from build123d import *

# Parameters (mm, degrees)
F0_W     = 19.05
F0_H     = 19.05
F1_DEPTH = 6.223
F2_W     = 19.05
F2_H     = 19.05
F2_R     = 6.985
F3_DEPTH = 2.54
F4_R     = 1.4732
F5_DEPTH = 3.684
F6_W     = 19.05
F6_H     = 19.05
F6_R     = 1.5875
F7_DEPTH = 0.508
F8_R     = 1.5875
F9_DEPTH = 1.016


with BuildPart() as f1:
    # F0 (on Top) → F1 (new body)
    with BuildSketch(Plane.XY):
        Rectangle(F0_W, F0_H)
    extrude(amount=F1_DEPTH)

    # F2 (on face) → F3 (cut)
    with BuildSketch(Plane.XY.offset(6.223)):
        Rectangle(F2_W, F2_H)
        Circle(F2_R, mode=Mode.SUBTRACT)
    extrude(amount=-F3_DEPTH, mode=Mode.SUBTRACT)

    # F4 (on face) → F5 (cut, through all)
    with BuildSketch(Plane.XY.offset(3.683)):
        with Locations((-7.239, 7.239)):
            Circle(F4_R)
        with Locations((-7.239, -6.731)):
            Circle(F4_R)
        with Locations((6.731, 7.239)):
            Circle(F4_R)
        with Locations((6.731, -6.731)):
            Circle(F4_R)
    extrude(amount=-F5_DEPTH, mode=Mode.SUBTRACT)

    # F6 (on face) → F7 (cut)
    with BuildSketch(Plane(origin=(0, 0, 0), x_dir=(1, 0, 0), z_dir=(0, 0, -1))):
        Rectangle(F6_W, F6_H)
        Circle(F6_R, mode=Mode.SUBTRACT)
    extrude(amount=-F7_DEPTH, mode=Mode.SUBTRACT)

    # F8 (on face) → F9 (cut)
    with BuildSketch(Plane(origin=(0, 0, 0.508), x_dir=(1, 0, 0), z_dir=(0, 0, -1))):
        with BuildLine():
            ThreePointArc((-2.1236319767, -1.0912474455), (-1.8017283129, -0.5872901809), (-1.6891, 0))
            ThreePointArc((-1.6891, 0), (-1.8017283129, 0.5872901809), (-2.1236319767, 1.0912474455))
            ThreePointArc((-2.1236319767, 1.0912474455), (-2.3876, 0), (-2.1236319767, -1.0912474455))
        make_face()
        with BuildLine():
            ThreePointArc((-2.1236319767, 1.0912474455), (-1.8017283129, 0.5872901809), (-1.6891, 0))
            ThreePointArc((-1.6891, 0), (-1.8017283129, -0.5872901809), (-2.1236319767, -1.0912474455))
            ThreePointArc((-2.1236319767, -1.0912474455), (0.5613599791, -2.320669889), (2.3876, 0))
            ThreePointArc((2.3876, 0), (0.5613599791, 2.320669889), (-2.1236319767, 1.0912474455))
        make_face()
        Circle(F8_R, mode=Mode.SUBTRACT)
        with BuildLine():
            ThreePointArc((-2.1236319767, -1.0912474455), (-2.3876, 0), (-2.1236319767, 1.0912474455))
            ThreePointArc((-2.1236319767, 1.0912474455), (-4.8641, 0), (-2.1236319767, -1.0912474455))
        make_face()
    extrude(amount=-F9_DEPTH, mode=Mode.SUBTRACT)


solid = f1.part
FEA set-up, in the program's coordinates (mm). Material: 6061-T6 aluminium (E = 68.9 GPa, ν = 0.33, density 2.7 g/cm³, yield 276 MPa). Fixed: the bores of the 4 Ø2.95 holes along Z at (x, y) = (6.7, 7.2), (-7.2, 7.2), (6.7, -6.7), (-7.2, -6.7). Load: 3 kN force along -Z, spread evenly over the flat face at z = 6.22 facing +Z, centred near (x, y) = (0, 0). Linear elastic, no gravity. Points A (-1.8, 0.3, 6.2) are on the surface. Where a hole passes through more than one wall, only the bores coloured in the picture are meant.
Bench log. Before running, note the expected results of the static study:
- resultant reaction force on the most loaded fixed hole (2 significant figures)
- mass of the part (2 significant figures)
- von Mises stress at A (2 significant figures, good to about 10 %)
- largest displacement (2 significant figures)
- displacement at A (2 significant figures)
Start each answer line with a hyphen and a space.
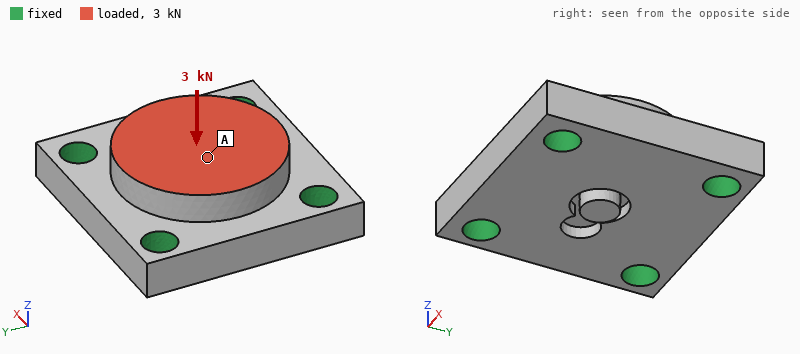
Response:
- 870 N
- 3.9 g
- 26 MPa
- 10 µm
- 10 µm
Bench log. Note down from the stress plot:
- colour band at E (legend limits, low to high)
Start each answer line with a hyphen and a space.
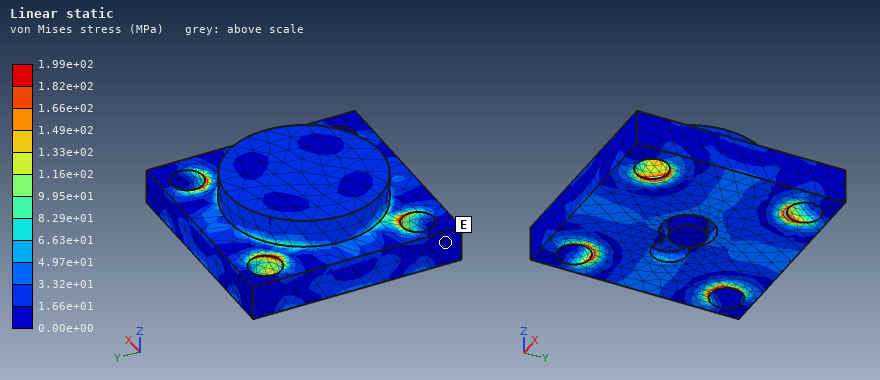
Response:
- 0.00e+00 to 1.66e+01 MPa
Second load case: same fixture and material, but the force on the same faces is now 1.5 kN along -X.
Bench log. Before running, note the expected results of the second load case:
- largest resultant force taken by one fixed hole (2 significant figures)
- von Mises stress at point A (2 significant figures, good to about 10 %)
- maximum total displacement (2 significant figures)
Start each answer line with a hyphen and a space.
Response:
- 500 N
- 17 MPa
- 5.7 µm
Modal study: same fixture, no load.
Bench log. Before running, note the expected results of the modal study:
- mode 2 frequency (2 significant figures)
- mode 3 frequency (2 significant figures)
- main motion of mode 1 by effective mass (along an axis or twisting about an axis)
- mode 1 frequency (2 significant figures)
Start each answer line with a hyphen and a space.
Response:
- 79 kHz
- 79 kHz
- along Z
- 58 kHz
